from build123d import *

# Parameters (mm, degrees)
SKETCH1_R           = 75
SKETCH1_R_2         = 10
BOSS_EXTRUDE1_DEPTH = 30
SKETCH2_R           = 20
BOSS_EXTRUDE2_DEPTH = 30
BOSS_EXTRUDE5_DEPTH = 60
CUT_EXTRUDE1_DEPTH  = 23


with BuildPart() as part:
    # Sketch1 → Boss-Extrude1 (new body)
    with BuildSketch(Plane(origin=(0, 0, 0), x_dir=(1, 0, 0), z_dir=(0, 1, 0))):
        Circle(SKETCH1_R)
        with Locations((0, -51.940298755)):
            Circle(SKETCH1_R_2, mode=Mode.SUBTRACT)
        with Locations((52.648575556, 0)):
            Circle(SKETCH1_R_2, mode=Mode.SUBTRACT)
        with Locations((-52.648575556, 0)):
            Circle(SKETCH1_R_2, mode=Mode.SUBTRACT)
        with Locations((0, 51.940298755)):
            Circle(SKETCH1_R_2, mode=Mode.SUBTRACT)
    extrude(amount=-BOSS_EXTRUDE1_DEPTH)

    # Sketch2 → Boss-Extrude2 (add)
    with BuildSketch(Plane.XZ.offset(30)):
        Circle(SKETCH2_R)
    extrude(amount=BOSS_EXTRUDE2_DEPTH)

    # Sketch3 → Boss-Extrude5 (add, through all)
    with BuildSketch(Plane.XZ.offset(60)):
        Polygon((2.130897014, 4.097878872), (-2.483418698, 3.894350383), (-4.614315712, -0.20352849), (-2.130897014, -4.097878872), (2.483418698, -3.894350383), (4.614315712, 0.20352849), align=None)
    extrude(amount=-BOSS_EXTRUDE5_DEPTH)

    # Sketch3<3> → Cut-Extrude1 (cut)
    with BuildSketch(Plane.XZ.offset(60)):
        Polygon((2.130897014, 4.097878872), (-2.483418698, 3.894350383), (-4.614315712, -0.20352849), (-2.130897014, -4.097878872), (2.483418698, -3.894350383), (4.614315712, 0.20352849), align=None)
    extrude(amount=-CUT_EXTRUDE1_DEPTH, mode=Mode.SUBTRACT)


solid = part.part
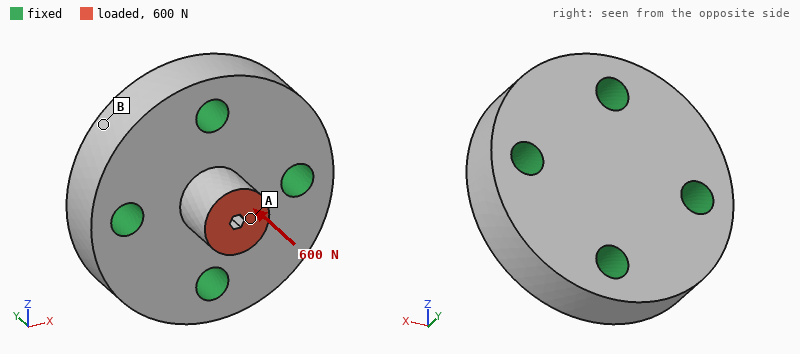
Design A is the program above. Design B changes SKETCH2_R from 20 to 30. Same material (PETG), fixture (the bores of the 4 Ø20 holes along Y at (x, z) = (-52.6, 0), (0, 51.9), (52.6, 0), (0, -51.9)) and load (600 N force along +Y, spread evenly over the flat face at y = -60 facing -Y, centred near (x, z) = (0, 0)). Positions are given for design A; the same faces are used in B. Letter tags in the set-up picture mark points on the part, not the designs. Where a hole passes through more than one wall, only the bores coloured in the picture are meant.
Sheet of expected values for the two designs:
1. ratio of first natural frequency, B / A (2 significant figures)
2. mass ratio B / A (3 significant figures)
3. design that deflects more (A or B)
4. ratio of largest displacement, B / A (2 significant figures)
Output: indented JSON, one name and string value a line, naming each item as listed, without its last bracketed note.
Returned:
{
  "ratio of first natural frequency, B / A": "1.00",
  "mass ratio B / A": "1.09",
  "design that deflects more": "A",
  "ratio of largest displacement, B / A": "0.51"
}
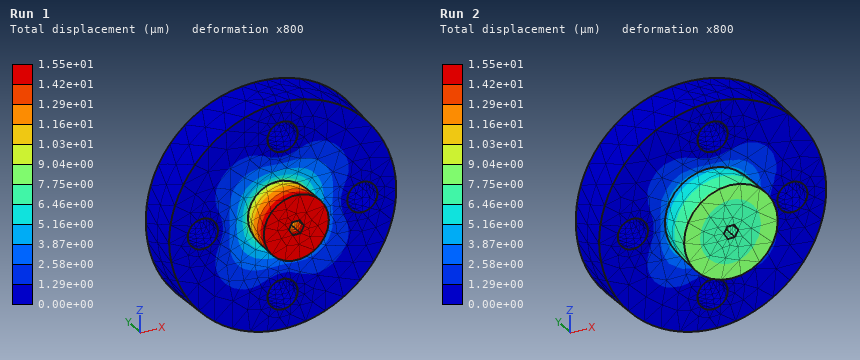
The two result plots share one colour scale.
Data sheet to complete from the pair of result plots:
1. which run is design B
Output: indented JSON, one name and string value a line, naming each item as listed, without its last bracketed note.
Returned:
{
  "which run is design B": "Run 2"
}
